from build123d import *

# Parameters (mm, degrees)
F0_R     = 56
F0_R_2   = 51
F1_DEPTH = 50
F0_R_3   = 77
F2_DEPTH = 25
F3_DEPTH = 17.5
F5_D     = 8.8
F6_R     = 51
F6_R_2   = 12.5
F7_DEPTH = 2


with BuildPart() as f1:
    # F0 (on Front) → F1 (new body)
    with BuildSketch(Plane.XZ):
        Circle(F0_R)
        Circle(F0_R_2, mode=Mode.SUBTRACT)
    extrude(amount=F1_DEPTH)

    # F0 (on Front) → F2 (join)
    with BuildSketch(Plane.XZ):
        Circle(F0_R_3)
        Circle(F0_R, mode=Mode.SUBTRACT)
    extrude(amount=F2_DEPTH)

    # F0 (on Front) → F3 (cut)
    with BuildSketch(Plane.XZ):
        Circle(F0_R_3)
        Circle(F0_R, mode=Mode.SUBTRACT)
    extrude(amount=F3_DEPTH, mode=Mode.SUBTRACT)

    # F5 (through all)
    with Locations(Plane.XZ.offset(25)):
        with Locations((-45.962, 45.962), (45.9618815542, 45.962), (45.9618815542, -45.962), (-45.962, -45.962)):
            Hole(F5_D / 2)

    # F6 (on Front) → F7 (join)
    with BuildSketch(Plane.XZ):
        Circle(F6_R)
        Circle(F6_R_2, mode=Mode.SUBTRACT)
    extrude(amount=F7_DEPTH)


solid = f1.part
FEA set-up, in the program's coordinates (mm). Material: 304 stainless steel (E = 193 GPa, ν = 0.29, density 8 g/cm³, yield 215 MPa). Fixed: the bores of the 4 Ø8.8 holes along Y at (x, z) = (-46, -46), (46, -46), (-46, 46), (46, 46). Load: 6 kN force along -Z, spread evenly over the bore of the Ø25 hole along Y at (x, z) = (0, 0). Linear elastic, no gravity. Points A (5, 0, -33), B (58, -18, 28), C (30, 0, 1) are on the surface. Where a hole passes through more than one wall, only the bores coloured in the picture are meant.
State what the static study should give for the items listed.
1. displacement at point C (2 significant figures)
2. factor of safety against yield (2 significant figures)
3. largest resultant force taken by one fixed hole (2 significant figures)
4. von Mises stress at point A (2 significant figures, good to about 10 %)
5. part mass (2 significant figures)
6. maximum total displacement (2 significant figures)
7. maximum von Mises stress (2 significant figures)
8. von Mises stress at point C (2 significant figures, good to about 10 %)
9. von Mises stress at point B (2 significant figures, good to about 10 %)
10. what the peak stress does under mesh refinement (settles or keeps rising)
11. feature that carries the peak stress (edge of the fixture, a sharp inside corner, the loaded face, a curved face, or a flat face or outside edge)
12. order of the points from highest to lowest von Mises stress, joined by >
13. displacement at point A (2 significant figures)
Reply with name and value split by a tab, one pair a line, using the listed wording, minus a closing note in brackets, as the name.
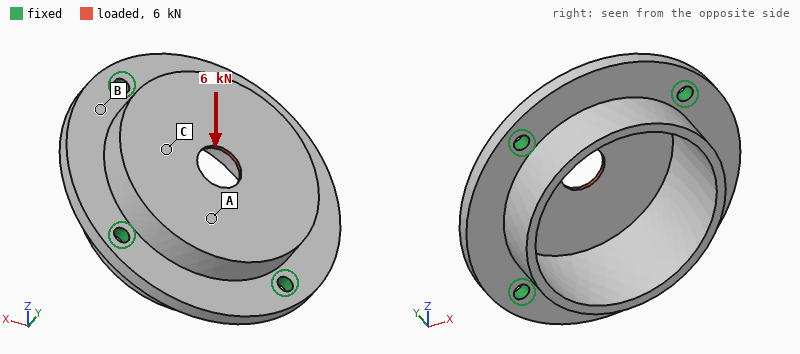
displacement at point C	7.8 µm
factor of safety against yield	3.1
largest resultant force taken by one fixed hole	1.7 kN
von Mises stress at point A	25 MPa
part mass	1.3 kg
maximum total displacement	15 µm
maximum von Mises stress	68 MPa
von Mises stress at point C	17 MPa
von Mises stress at point B	5.2 MPa
what the peak stress does under mesh refinement	settles
feature that carries the peak stress	the loaded face
order of the points from highest to lowest von Mises stress, joined by >	A > C > B
displacement at point A	13 µm
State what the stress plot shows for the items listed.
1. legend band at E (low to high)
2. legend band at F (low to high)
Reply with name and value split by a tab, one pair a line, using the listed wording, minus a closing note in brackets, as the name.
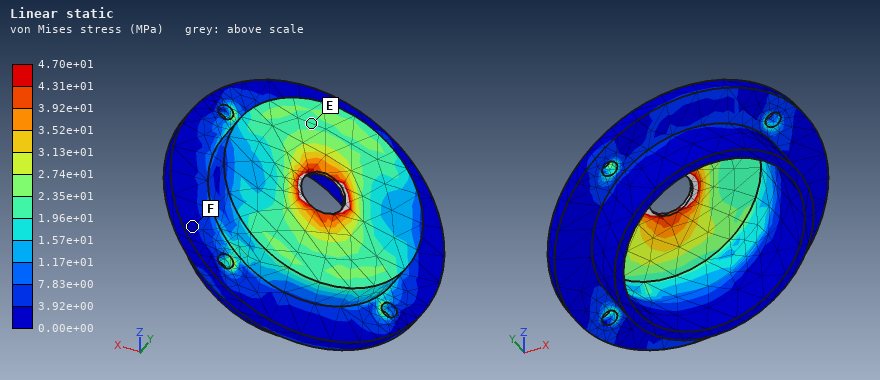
legend band at E	1.96e+01 to 2.35e+01 MPa
legend band at F	0.00e+00 to 3.92e+00 MPa
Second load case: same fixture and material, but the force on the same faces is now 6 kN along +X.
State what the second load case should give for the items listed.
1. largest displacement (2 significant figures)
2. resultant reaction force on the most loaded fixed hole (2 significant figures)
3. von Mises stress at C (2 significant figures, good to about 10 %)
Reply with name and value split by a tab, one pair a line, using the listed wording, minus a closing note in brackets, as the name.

largest displacement	15 µm
resultant reaction force on the most loaded fixed hole	1.7 kN
von Mises stress at C	27 MPa
